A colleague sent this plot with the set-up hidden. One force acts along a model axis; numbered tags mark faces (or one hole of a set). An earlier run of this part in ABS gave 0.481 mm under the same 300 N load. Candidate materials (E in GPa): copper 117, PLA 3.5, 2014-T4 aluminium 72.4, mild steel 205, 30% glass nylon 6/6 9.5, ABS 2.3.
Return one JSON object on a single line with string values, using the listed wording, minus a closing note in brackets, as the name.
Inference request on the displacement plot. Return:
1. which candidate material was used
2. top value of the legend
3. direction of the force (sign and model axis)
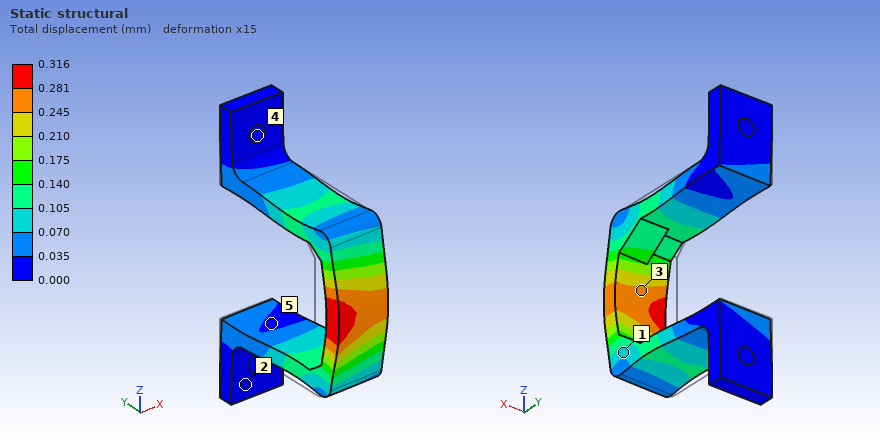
{"which candidate material was used": "PLA", "top value of the legend": "0.316 mm", "direction of the force": "-Y"}
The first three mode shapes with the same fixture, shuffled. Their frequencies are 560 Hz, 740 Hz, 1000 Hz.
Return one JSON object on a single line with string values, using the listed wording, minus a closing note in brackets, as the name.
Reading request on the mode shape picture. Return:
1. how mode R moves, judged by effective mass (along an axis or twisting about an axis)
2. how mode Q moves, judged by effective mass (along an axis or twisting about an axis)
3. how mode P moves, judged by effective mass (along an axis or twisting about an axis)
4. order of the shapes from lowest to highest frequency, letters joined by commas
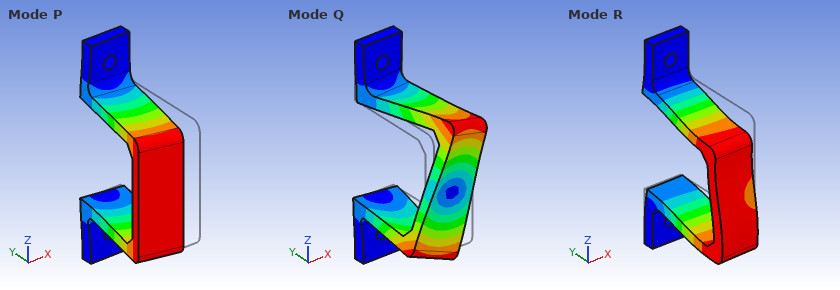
{"how mode R moves, judged by effective mass": "along Z", "how mode Q moves, judged by effective mass": "twisting about Y", "how mode P moves, judged by effective mass": "along X", "order of the shapes from lowest to highest frequency, letters joined by commas": "P, R, Q"}
